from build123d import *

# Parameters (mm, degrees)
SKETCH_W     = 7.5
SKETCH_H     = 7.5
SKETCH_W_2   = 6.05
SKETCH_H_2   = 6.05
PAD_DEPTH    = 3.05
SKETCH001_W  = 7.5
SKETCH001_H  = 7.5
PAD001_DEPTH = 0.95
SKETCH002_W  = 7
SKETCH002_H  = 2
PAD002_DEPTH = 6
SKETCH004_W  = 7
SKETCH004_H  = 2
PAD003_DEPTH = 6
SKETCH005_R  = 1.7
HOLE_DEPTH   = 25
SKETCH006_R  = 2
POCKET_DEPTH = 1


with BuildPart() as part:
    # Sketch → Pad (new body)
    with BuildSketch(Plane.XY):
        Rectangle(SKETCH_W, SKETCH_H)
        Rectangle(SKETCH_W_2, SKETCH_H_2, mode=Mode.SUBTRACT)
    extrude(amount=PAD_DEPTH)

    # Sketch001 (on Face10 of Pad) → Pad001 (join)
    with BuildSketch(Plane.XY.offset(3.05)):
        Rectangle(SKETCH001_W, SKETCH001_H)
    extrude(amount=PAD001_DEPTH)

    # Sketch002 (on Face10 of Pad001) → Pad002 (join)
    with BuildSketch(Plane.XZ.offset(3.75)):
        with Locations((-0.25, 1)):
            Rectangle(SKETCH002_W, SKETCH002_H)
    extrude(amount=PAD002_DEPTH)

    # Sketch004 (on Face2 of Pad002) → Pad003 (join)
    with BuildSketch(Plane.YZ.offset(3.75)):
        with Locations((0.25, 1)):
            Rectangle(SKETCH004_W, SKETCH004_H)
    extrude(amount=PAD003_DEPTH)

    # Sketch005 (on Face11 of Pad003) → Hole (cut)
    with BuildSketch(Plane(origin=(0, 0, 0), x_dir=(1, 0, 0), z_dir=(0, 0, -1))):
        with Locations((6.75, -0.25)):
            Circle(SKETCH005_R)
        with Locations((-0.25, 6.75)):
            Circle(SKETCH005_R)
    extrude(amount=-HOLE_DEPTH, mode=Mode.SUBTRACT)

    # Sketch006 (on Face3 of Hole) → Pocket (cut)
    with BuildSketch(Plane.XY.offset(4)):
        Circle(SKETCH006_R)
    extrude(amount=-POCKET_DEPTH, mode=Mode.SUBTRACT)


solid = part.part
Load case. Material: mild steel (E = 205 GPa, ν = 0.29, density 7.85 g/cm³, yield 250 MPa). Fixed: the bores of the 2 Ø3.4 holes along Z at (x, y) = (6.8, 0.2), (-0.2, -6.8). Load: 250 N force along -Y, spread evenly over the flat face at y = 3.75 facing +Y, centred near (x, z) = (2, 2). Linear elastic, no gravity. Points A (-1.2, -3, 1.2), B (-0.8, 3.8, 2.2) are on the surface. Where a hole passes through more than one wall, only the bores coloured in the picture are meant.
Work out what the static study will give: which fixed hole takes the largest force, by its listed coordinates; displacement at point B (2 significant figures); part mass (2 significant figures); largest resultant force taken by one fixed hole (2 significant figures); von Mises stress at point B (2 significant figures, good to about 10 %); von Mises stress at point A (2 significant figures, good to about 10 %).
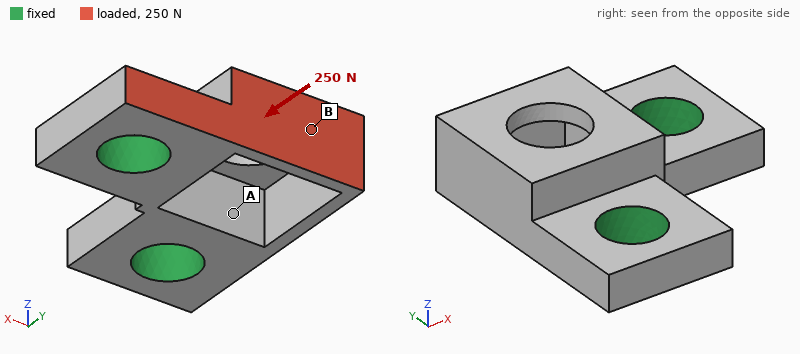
(6.8, 0.2)
3.7 µm
1.8 g
150 N
60 MPa
20 MPa
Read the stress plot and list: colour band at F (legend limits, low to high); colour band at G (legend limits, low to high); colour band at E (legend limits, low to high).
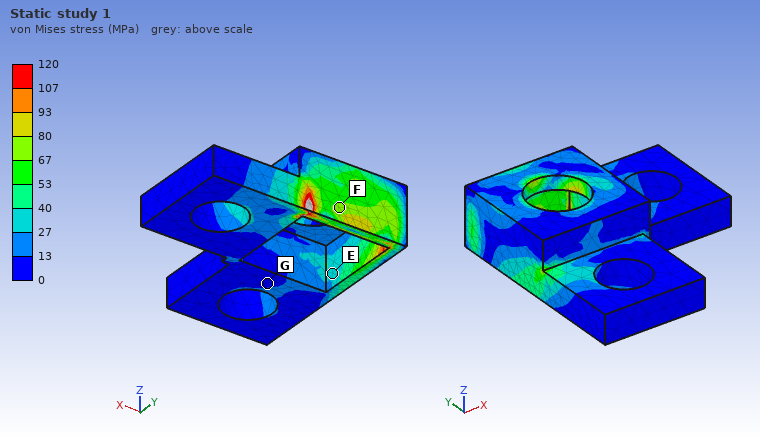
67 to 80 MPa
0 to 13 MPa
27 to 40 MPa
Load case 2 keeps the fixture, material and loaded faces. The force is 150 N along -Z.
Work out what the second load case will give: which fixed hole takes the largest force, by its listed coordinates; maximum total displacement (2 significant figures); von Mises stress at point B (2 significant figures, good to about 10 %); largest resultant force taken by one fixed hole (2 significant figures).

(6.8, 0.2)
13 µm
32 MPa
140 N
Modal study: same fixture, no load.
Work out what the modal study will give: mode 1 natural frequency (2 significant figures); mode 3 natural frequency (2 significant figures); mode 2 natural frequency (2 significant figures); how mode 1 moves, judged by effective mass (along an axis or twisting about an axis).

29 kHz
87 kHz
63 kHz
along Z
